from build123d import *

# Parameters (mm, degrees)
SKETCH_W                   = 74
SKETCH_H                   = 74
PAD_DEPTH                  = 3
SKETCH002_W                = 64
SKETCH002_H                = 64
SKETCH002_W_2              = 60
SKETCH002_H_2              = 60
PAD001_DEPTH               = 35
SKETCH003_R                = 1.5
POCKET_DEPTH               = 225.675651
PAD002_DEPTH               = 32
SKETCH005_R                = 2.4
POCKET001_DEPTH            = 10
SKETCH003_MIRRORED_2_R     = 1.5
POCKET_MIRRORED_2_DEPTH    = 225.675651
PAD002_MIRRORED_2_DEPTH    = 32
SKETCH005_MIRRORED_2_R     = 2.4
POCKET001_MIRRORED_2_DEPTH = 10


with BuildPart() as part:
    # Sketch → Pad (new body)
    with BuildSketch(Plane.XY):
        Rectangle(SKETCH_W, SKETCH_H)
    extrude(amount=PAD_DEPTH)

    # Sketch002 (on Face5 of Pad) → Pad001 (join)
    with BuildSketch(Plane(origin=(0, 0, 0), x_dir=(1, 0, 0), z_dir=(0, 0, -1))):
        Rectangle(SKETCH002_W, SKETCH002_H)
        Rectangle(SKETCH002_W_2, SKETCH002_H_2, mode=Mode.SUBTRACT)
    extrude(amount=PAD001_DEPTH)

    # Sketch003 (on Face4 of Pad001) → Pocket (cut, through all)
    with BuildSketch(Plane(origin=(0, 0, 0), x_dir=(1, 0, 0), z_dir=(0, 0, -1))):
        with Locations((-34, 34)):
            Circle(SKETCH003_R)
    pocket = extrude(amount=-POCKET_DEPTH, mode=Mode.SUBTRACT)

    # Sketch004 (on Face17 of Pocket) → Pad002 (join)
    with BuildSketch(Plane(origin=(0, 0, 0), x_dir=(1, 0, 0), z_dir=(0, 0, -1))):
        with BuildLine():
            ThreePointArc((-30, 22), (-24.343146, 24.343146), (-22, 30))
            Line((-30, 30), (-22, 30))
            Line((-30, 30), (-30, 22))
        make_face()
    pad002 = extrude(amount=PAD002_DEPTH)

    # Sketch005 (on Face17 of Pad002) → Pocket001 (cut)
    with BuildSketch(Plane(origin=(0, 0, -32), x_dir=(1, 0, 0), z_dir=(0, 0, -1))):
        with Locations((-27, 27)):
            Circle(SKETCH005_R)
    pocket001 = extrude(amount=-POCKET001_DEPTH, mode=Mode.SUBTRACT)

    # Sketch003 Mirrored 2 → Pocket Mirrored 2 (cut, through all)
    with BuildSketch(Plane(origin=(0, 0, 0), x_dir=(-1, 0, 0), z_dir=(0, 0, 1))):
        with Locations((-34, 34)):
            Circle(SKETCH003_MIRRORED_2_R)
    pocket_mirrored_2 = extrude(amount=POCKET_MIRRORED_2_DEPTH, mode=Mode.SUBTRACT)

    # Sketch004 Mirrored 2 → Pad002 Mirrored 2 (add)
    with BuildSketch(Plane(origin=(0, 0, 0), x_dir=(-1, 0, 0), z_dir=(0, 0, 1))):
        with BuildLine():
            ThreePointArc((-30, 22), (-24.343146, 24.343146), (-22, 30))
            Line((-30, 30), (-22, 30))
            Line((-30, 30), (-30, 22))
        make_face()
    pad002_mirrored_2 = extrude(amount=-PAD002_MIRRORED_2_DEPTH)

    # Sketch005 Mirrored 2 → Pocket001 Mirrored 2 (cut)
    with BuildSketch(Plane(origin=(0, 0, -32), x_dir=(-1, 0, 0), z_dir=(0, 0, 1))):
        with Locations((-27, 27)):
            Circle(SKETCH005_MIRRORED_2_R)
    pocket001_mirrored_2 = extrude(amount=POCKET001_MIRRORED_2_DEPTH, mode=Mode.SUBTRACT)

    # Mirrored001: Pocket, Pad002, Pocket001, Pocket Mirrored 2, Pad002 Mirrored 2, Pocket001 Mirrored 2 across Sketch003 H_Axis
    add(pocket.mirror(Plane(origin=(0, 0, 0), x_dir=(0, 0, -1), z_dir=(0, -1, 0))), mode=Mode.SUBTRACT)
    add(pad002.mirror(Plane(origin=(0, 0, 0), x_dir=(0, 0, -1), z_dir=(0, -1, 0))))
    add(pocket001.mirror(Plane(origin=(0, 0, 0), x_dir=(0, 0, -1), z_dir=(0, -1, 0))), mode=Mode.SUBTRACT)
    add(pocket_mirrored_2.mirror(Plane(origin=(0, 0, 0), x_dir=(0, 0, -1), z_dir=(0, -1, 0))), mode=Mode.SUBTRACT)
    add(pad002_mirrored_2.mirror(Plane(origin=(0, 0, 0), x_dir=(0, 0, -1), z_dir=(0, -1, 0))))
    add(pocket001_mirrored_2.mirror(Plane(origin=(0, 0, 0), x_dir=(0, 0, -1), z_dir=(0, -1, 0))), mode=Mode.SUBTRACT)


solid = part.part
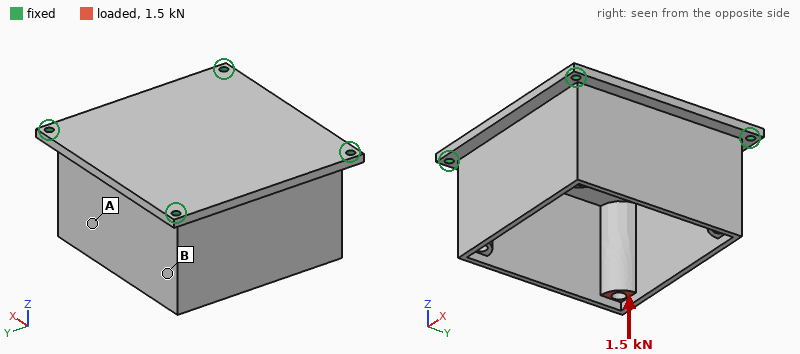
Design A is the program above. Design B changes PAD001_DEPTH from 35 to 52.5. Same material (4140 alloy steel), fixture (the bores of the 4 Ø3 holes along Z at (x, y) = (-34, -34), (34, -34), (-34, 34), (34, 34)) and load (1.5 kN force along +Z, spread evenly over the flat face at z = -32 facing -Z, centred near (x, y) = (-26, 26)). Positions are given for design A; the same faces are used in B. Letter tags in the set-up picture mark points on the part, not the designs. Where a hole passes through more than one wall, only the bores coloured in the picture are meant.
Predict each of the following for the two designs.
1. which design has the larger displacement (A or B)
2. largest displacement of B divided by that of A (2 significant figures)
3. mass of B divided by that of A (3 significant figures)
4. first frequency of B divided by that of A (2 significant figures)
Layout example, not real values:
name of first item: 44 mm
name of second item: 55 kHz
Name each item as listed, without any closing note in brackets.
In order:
which design has the larger displacement: B
largest displacement of B divided by that of A: 1.3
mass of B divided by that of A: 1.22
first frequency of B divided by that of A: 0.62
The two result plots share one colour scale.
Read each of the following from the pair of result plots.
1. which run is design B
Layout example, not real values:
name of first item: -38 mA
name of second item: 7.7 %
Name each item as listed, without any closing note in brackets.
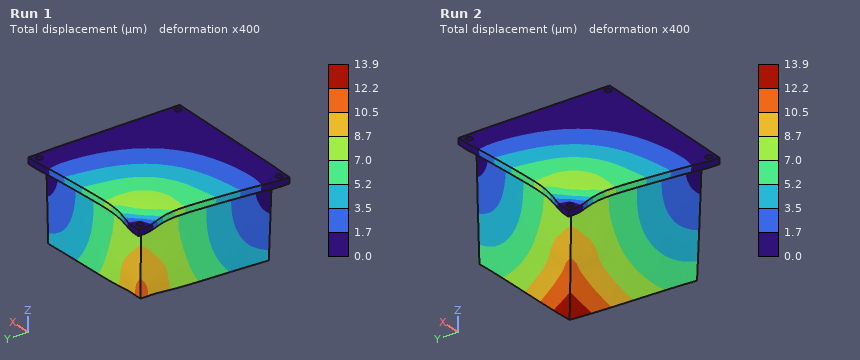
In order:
which run is design B: Run 2
